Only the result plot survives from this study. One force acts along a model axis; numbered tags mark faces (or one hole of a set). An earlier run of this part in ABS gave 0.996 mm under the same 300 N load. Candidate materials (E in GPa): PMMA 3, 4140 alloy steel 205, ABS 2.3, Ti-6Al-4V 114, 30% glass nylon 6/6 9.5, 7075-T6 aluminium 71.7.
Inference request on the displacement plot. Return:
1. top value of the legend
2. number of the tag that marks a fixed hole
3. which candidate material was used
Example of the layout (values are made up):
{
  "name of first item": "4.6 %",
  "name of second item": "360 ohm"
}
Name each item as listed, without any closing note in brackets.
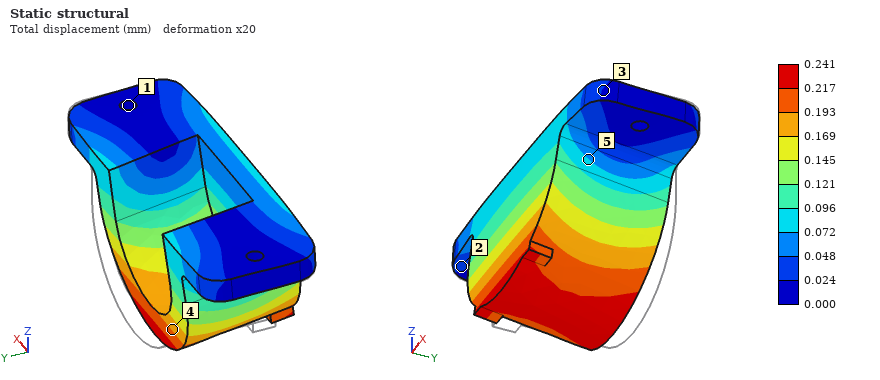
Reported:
{
  "top value of the legend": "0.241 mm",
  "number of the tag that marks a fixed hole": "1",
  "which candidate material was used": "30% glass nylon 6/6"
}
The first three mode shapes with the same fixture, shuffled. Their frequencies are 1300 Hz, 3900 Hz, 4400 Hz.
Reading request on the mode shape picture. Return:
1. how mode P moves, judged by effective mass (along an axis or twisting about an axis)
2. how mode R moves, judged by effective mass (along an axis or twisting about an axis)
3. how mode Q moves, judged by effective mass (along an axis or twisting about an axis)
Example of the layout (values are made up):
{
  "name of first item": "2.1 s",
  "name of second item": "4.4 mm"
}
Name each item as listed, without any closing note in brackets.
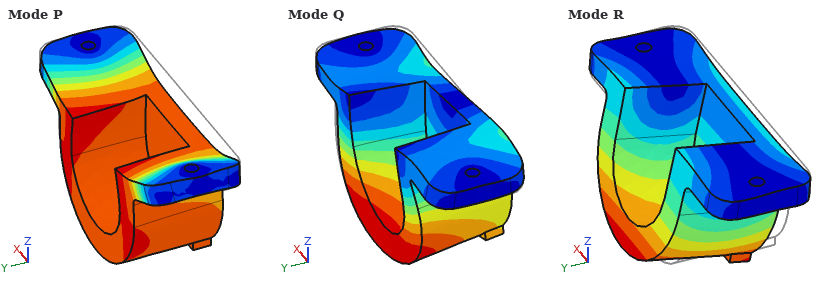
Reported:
{
  "how mode P moves, judged by effective mass": "along Z",
  "how mode R moves, judged by effective mass": "along Y",
  "how mode Q moves, judged by effective mass": "along X"
}
